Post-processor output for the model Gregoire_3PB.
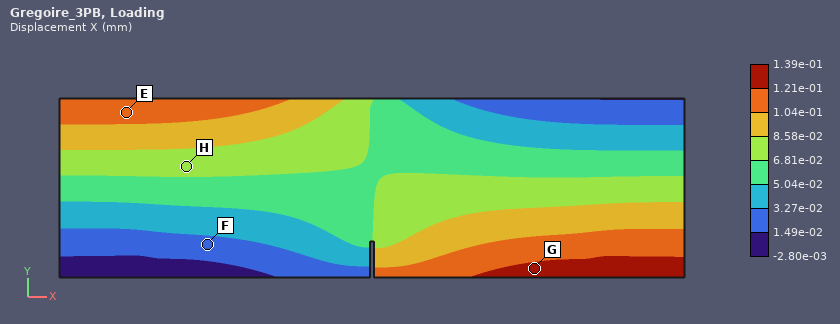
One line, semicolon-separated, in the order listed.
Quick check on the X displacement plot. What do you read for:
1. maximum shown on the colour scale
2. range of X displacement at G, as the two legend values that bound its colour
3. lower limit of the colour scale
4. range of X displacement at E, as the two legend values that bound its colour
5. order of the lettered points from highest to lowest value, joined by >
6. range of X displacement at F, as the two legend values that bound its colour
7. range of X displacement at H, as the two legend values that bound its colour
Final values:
1.39e-01 mm; 1.21e-01 to 1.39e-01 mm; -2.80e-03 mm; 1.04e-01 to 1.21e-01 mm; G > E > H > F; 1.49e-02 to 3.27e-02 mm; 6.81e-02 to 8.58e-02 mm
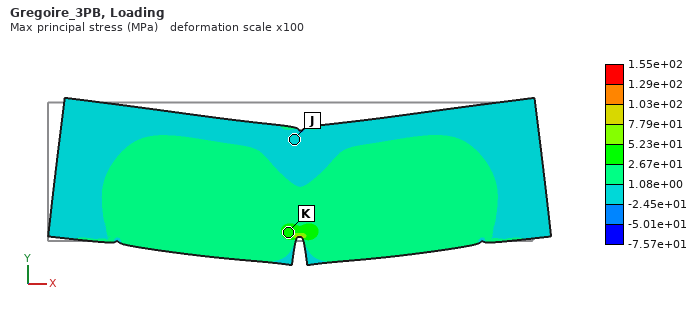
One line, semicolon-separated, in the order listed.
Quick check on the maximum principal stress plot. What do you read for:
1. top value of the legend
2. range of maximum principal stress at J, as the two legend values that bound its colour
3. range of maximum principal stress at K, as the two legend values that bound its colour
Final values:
1.55e+02 MPa; -2.45e+01 to 1.08e+00 MPa; 2.67e+01 to 5.23e+01 MPa
